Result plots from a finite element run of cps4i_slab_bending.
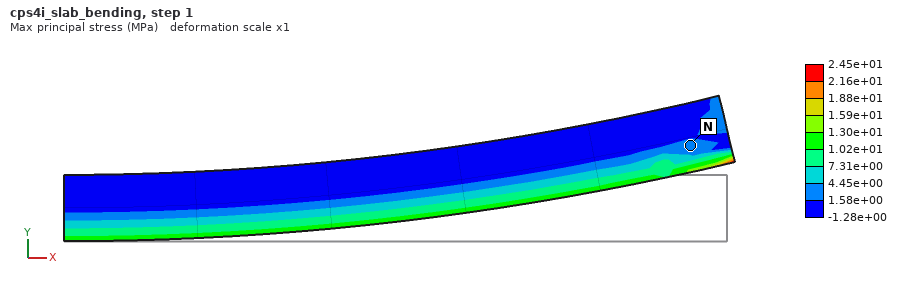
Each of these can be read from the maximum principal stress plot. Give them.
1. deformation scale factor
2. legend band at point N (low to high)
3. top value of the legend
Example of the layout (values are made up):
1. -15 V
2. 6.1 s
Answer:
1. 1
2. 1.58e+00 to 4.45e+00 MPa
3. 2.45e+01 MPa
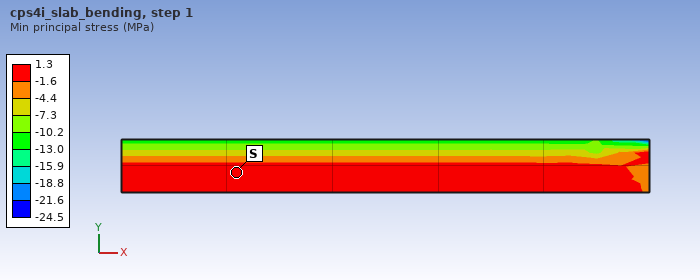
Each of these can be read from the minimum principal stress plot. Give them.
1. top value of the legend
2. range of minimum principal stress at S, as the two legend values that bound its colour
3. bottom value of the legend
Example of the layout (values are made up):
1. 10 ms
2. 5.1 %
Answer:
1. 1.3 MPa
2. -1.6 to 1.3 MPa
3. -24.5 MPa
